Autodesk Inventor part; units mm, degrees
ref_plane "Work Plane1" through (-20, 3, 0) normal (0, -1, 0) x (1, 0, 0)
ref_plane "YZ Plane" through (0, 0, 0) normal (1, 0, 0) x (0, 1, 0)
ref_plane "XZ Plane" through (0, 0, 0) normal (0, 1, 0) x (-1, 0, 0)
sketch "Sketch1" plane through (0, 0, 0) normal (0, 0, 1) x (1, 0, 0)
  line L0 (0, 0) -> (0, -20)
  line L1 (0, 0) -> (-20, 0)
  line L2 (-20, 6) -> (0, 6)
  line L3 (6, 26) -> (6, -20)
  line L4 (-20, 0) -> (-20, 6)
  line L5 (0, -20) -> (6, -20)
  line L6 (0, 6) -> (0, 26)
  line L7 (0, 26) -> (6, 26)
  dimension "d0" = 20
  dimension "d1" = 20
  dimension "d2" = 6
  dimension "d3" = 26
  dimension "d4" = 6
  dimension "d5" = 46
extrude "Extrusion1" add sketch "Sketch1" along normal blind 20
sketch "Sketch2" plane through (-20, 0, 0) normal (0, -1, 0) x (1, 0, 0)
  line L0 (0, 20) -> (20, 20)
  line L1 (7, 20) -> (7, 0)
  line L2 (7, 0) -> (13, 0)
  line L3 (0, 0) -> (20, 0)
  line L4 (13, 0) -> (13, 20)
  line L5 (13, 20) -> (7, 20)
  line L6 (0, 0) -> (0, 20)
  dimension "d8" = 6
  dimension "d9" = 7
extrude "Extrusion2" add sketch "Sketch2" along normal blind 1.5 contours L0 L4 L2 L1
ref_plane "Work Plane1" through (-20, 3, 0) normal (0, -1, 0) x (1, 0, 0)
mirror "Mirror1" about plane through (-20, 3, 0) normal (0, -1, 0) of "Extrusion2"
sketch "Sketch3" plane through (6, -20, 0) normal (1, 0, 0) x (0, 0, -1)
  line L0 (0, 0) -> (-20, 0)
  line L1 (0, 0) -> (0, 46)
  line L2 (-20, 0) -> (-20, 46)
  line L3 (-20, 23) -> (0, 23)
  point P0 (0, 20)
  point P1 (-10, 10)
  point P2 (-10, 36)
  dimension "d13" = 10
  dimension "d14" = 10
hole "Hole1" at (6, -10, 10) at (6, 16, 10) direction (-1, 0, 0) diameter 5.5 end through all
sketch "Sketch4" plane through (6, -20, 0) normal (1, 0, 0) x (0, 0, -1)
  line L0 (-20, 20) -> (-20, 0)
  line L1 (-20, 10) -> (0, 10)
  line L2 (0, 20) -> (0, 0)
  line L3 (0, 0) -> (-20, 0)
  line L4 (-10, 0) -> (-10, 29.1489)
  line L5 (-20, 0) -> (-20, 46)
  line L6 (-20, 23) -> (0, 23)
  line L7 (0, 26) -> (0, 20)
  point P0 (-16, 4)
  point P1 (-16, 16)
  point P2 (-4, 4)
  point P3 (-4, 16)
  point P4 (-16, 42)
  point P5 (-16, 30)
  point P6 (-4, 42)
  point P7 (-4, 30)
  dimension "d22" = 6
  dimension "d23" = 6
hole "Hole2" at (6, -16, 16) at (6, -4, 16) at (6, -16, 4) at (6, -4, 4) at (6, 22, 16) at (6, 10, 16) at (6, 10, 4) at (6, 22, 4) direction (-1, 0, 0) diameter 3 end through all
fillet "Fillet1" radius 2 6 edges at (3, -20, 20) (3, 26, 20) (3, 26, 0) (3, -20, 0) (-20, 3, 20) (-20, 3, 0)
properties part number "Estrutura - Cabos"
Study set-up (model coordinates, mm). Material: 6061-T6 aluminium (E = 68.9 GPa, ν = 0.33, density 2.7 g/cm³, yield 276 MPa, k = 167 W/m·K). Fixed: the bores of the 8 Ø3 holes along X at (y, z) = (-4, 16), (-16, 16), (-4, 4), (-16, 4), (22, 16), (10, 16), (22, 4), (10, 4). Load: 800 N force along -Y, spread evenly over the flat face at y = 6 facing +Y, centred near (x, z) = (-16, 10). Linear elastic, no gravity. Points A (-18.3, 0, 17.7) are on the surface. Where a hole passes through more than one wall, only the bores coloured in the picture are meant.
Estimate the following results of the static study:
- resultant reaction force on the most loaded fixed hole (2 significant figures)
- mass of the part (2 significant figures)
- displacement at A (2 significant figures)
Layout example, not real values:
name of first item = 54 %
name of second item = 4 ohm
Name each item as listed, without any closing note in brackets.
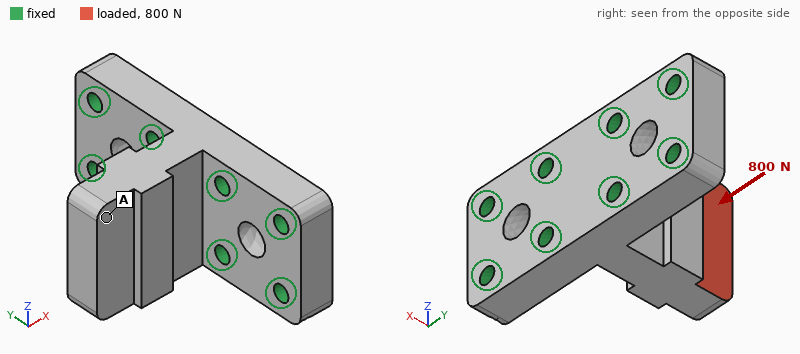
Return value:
resultant reaction force on the most loaded fixed hole = 680 N
mass of the part = 21 g
displacement at A = 76 µm
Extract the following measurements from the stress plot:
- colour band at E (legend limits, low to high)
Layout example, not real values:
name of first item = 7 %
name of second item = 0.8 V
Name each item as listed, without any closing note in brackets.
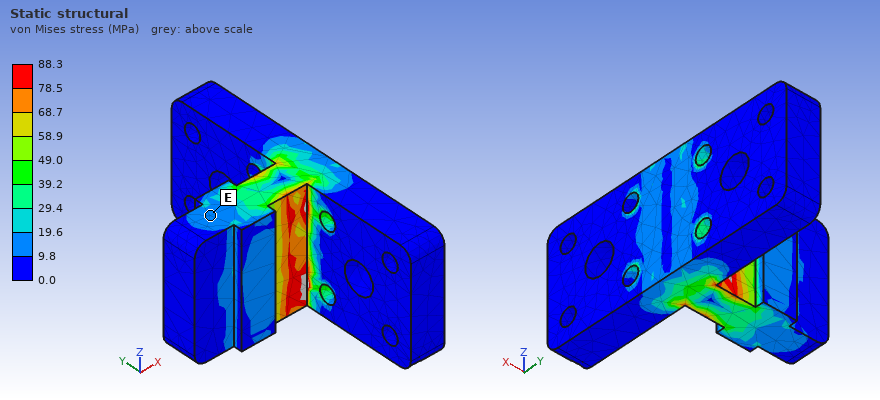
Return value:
colour band at E = 9.8 to 19.6 MPa
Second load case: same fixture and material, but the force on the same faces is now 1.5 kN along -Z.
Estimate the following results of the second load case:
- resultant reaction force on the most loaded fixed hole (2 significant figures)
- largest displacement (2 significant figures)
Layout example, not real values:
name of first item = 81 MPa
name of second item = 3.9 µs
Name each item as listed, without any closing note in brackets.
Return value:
resultant reaction force on the most loaded fixed hole = 1.2 kN
largest displacement = 49 µm
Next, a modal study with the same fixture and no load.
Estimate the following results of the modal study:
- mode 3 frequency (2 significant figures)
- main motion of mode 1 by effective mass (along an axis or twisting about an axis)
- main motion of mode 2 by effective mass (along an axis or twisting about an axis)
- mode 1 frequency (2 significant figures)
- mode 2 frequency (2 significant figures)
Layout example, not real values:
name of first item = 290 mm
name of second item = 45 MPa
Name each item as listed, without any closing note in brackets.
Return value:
mode 3 frequency = 23 kHz
main motion of mode 1 by effective mass = along Y
main motion of mode 2 by effective mass = along Z
mode 1 frequency = 9500 Hz
mode 2 frequency = 16 kHz
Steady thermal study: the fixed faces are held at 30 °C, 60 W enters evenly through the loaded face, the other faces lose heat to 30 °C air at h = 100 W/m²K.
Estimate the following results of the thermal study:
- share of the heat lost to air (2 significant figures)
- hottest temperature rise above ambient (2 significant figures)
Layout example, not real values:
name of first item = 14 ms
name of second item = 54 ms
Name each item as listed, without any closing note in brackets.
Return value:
share of the heat lost to air = 7.3 %
hottest temperature rise above ambient = 58 K
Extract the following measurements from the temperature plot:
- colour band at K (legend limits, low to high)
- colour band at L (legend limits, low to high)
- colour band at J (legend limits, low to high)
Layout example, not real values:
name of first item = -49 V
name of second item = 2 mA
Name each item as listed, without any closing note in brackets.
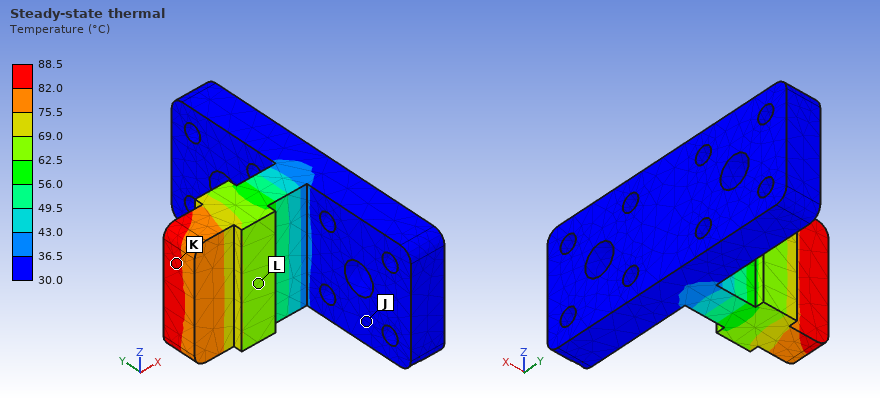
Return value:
colour band at K = 82.0 to 88.5 °C
colour band at L = 62.5 to 69.0 °C
colour band at J = 30.0 to 36.5 °C
